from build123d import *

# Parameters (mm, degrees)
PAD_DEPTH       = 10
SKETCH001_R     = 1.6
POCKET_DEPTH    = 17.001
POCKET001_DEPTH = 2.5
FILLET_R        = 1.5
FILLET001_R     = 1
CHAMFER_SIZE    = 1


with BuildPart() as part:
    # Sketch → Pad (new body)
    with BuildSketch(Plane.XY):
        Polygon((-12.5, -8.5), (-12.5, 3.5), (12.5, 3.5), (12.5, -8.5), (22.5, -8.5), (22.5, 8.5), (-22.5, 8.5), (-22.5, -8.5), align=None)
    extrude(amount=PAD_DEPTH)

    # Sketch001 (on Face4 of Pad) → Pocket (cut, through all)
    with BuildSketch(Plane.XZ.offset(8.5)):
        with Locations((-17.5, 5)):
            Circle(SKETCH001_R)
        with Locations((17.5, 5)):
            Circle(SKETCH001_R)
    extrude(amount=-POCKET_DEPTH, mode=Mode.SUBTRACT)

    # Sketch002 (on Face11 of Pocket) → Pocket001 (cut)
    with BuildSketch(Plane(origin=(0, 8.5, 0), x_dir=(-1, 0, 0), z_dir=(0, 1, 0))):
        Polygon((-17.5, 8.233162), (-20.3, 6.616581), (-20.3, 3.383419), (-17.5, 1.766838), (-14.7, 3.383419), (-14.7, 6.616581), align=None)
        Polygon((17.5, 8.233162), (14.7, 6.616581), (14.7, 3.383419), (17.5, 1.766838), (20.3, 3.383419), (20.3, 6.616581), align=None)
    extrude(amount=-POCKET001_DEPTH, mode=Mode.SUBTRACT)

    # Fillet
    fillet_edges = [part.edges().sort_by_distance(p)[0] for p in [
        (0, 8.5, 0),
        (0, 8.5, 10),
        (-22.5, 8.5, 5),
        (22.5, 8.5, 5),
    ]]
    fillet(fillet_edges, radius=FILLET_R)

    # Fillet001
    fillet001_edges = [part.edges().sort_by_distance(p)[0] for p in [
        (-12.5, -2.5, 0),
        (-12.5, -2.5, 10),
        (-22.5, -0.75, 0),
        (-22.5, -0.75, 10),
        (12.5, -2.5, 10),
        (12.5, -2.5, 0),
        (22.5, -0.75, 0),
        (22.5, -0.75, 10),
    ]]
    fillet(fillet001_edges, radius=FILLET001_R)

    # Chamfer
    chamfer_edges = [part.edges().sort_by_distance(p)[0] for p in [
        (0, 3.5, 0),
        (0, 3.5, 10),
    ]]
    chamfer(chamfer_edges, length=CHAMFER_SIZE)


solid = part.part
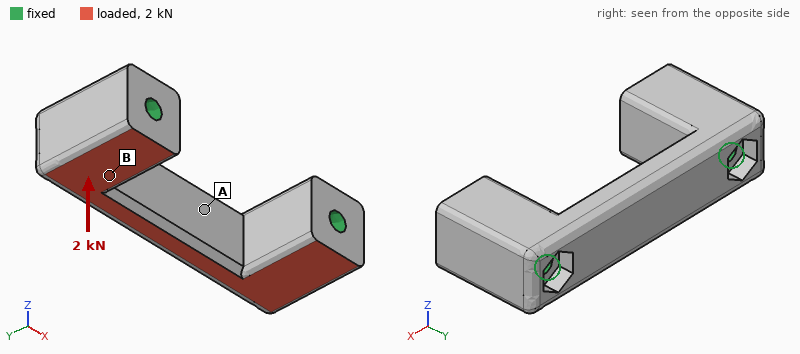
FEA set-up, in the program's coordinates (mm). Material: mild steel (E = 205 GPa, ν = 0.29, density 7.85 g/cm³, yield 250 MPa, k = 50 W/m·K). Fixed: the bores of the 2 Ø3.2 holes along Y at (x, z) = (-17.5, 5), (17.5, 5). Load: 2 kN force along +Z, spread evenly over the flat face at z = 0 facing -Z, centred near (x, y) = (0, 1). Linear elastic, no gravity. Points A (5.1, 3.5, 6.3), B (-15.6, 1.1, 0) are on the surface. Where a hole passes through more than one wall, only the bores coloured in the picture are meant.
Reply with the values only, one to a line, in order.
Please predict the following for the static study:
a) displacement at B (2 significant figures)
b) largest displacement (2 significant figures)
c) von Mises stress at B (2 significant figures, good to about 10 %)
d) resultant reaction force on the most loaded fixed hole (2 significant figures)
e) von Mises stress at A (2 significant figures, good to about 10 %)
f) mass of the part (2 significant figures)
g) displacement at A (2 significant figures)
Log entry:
0.34 µm
1.9 µm
12 MPa
1.0 kN
5.3 MPa
33 g
1.5 µm
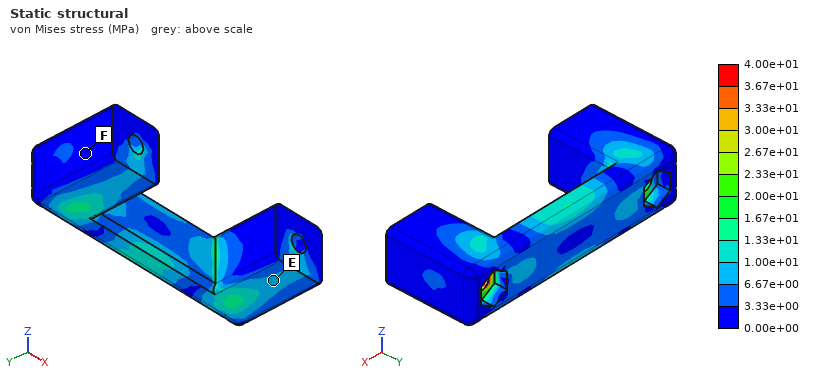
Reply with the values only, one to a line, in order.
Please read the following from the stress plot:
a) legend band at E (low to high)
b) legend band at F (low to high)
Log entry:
6.67e+00 to 1.00e+01 MPa
0.00e+00 to 3.33e+00 MPa
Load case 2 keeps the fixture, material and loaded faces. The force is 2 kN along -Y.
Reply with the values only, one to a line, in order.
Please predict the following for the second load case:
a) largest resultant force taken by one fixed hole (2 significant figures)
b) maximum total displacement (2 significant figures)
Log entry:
1.0 kN
5.0 µm
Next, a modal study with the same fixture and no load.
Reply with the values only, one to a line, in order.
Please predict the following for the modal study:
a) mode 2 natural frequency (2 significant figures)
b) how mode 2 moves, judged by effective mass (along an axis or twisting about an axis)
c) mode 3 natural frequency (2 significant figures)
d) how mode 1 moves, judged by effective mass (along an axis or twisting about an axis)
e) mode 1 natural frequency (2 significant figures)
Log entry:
27 kHz
along Z
42 kHz
along Y
23 kHz
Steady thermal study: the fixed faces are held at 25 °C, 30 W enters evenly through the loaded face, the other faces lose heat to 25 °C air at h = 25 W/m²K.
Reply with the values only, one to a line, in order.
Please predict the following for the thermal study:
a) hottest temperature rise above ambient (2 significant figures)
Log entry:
20 K
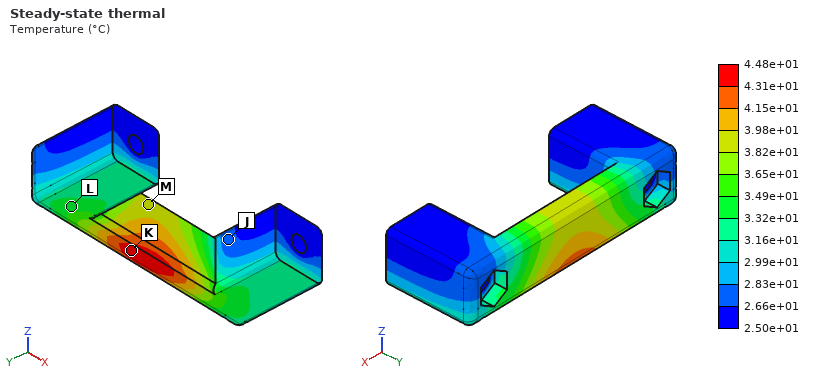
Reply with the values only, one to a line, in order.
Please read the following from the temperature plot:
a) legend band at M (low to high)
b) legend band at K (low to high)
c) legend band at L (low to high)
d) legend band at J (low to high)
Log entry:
3.82e+01 to 3.98e+01 °C
4.31e+01 to 4.48e+01 °C
3.32e+01 to 3.49e+01 °C
2.66e+01 to 2.83e+01 °C
